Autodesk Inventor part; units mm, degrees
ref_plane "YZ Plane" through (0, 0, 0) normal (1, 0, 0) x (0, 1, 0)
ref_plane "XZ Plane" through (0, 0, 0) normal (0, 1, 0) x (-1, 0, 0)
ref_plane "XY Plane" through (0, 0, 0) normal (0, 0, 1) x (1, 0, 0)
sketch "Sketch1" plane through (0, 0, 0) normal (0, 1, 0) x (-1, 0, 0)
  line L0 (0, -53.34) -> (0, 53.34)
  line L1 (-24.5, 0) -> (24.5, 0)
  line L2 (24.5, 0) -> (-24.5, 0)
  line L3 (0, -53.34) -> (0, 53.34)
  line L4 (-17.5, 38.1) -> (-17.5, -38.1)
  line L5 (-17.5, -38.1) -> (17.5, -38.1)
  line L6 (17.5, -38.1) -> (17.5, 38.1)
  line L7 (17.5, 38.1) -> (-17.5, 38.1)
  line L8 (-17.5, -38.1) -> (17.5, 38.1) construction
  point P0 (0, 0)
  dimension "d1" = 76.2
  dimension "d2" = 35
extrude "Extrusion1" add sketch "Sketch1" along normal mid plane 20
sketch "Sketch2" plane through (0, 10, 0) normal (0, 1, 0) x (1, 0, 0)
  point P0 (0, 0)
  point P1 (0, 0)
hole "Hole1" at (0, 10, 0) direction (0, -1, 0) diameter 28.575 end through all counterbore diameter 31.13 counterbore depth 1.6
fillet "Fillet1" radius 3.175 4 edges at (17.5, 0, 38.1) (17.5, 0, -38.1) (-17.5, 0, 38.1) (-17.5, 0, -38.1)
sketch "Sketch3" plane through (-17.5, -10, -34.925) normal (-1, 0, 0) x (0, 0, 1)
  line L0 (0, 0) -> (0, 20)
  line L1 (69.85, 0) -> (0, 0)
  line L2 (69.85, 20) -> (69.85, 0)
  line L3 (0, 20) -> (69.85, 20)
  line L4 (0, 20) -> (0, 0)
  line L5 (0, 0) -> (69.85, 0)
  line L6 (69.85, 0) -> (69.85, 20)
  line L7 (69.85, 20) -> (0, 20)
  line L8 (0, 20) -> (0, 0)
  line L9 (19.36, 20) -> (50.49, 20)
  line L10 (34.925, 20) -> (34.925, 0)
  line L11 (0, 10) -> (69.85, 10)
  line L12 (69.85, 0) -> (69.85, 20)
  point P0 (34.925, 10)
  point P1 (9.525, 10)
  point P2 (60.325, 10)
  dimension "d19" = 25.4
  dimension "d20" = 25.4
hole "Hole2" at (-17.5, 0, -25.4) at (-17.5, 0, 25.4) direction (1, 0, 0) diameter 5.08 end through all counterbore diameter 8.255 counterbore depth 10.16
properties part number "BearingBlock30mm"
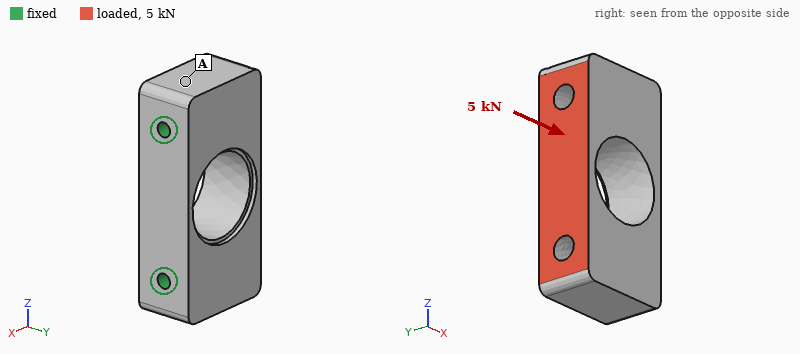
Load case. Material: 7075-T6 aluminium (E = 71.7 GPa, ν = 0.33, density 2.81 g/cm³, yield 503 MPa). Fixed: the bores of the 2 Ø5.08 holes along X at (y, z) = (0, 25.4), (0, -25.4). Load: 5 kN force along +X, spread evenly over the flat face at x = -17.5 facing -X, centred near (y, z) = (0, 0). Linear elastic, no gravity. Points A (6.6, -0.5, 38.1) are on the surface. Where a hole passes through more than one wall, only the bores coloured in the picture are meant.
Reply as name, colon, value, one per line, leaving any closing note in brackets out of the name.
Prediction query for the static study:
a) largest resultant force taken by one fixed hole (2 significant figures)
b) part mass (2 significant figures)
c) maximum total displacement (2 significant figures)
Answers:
largest resultant force taken by one fixed hole: 2.6 kN
part mass: 110 g
maximum total displacement: 12 µm
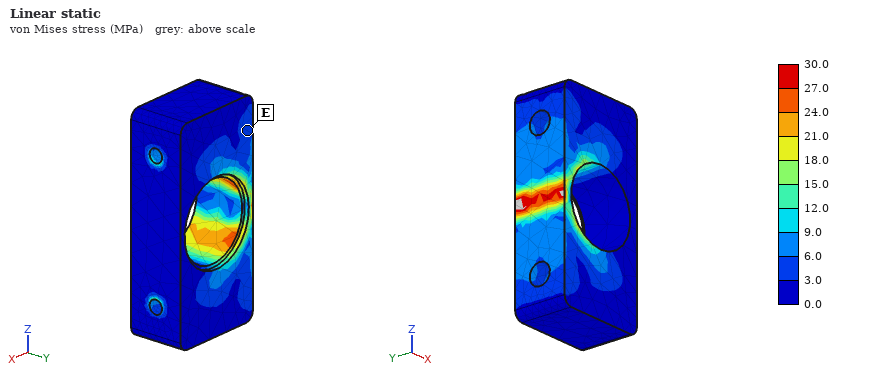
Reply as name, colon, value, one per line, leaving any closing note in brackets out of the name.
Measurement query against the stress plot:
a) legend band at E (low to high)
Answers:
legend band at E: 3.0 to 6.0 MPa
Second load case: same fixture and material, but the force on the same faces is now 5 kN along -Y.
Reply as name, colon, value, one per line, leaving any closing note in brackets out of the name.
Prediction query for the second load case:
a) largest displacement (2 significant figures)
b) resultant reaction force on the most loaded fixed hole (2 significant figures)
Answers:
largest displacement: 31 µm
resultant reaction force on the most loaded fixed hole: 2.5 kN
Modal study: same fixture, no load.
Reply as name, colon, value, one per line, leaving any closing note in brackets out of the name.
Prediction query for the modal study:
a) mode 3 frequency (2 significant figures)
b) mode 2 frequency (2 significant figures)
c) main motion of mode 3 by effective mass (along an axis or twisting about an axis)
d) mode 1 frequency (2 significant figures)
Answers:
mode 3 frequency: 23 kHz
mode 2 frequency: 21 kHz
main motion of mode 3 by effective mass: along Z
mode 1 frequency: 17 kHz
